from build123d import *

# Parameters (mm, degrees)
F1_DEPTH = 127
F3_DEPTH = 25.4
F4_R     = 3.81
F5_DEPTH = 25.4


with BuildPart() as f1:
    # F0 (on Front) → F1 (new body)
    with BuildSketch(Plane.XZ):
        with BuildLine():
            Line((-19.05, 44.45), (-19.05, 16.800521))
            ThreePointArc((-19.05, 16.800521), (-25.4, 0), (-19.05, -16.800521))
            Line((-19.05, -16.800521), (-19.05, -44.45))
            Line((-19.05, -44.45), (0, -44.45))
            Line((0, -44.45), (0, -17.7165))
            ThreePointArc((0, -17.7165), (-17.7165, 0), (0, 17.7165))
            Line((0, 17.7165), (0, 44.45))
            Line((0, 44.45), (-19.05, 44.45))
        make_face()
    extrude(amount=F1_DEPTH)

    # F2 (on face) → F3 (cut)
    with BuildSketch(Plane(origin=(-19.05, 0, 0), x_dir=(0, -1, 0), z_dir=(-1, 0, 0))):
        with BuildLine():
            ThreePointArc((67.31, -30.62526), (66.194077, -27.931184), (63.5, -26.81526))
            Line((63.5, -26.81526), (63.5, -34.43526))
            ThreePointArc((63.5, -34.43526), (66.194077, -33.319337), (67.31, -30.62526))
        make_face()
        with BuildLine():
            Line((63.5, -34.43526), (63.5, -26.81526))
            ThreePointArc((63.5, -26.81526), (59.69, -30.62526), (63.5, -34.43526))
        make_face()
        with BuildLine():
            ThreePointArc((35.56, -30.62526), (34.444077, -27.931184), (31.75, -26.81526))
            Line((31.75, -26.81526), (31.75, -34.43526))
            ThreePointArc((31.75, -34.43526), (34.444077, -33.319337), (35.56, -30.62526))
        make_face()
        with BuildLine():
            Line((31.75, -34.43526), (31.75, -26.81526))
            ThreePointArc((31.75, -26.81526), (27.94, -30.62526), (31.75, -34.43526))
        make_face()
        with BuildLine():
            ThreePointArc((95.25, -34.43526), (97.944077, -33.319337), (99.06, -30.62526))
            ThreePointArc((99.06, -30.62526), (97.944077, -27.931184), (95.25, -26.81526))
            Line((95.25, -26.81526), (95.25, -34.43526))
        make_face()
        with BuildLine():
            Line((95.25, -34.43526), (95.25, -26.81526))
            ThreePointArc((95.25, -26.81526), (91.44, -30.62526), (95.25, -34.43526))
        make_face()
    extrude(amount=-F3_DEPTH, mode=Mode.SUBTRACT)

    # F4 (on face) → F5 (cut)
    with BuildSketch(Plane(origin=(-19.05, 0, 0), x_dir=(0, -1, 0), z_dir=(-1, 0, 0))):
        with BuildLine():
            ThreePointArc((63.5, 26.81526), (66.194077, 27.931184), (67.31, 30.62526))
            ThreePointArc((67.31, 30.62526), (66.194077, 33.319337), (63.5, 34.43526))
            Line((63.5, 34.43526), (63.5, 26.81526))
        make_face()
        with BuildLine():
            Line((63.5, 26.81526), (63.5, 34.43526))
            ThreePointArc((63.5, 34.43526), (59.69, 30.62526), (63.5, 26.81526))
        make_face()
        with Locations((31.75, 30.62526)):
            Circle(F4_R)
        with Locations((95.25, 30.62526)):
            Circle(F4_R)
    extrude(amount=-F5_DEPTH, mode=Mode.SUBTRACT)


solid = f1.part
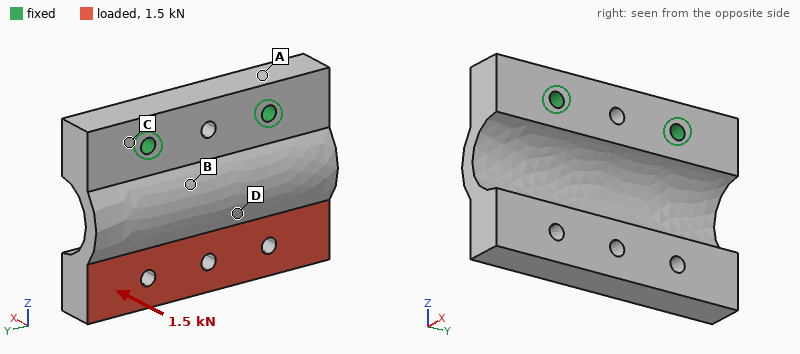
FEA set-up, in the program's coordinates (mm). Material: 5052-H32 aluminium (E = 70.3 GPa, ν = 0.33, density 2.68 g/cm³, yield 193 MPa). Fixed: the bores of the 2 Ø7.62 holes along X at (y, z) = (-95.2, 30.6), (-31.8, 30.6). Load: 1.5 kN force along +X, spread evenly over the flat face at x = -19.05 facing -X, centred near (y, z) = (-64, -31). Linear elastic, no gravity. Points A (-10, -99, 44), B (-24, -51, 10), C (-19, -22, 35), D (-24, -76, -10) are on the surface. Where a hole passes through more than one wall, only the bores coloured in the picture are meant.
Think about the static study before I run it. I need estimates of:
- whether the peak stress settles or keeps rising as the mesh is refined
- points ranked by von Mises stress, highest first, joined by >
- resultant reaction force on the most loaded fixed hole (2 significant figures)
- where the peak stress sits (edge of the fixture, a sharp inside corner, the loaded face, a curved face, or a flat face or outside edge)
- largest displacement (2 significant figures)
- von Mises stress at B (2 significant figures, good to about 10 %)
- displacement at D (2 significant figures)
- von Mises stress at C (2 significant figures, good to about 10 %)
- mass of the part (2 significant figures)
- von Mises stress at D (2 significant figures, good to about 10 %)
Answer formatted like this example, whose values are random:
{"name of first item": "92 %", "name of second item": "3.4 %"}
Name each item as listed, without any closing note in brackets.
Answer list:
{"whether the peak stress settles or keeps rising as the mesh is refined": "keeps rising", "points ranked by von Mises stress, highest first, joined by >": "B > D > C > A", "resultant reaction force on the most loaded fixed hole": "750 N", "where the peak stress sits": "edge of the fixture", "largest displacement": "0.28 mm", "von Mises stress at B": "36 MPa", "displacement at D": "0.087 mm", "von Mises stress at C": "9.3 MPa", "mass of the part": "440 g", "von Mises stress at D": "23 MPa"}
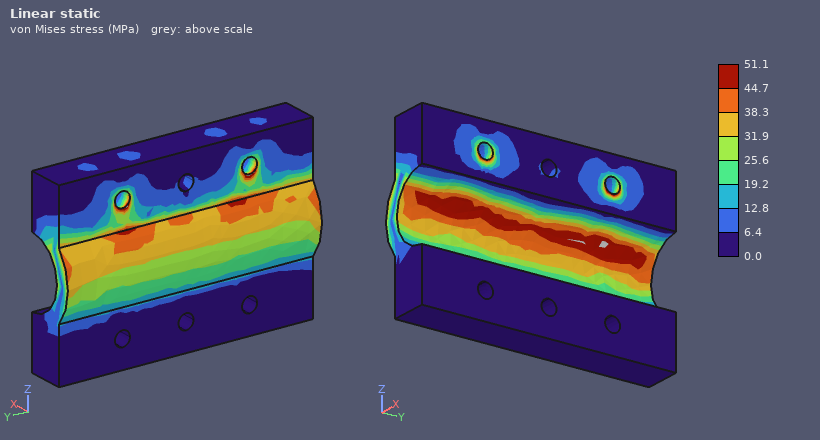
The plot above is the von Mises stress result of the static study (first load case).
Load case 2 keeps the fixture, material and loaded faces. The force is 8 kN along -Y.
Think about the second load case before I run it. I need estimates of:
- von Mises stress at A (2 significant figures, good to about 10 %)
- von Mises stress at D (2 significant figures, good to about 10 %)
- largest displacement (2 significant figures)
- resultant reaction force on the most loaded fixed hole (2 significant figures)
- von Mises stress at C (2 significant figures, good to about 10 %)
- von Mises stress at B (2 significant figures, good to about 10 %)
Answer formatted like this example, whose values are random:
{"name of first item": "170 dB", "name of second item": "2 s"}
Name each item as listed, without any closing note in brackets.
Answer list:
{"von Mises stress at A": "20 MPa", "von Mises stress at D": "21 MPa", "largest displacement": "72 µm", "resultant reaction force on the most loaded fixed hole": "8.0 kN", "von Mises stress at C": "22 MPa", "von Mises stress at B": "13 MPa"}
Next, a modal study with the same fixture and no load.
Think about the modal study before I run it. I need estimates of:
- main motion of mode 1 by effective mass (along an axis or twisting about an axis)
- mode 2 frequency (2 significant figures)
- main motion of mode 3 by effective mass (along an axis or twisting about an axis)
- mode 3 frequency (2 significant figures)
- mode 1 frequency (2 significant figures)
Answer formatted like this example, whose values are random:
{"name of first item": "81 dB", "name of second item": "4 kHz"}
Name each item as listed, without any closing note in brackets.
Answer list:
{"main motion of mode 1 by effective mass": "along X", "mode 2 frequency": "2200 Hz", "main motion of mode 3 by effective mass": "along Y", "mode 3 frequency": "4100 Hz", "mode 1 frequency": "980 Hz"}
